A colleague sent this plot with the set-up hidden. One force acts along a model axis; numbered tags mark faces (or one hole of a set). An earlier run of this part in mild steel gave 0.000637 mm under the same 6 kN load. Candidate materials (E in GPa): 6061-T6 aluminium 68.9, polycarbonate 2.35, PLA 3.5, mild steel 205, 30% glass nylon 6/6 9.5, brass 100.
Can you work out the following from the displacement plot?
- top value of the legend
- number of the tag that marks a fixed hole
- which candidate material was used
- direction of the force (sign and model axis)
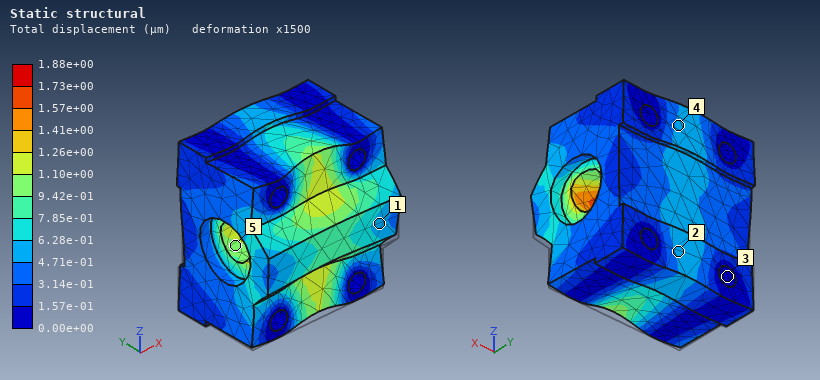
1.88e+00 µm
3
6061-T6 aluminium
+Z
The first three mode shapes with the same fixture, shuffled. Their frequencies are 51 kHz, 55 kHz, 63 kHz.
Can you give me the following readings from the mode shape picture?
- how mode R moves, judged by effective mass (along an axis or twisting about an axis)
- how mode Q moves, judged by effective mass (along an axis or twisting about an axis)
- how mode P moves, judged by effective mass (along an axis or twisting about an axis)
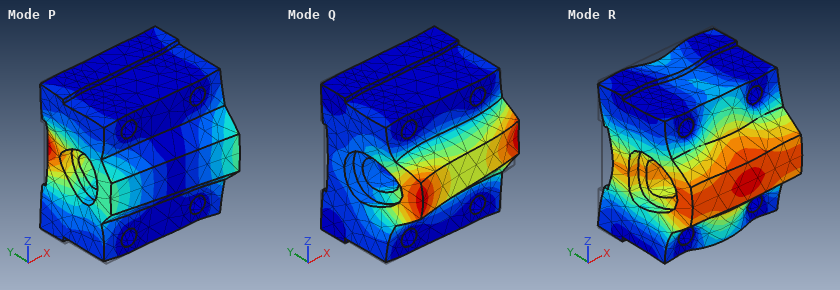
along Y
along X
along X
